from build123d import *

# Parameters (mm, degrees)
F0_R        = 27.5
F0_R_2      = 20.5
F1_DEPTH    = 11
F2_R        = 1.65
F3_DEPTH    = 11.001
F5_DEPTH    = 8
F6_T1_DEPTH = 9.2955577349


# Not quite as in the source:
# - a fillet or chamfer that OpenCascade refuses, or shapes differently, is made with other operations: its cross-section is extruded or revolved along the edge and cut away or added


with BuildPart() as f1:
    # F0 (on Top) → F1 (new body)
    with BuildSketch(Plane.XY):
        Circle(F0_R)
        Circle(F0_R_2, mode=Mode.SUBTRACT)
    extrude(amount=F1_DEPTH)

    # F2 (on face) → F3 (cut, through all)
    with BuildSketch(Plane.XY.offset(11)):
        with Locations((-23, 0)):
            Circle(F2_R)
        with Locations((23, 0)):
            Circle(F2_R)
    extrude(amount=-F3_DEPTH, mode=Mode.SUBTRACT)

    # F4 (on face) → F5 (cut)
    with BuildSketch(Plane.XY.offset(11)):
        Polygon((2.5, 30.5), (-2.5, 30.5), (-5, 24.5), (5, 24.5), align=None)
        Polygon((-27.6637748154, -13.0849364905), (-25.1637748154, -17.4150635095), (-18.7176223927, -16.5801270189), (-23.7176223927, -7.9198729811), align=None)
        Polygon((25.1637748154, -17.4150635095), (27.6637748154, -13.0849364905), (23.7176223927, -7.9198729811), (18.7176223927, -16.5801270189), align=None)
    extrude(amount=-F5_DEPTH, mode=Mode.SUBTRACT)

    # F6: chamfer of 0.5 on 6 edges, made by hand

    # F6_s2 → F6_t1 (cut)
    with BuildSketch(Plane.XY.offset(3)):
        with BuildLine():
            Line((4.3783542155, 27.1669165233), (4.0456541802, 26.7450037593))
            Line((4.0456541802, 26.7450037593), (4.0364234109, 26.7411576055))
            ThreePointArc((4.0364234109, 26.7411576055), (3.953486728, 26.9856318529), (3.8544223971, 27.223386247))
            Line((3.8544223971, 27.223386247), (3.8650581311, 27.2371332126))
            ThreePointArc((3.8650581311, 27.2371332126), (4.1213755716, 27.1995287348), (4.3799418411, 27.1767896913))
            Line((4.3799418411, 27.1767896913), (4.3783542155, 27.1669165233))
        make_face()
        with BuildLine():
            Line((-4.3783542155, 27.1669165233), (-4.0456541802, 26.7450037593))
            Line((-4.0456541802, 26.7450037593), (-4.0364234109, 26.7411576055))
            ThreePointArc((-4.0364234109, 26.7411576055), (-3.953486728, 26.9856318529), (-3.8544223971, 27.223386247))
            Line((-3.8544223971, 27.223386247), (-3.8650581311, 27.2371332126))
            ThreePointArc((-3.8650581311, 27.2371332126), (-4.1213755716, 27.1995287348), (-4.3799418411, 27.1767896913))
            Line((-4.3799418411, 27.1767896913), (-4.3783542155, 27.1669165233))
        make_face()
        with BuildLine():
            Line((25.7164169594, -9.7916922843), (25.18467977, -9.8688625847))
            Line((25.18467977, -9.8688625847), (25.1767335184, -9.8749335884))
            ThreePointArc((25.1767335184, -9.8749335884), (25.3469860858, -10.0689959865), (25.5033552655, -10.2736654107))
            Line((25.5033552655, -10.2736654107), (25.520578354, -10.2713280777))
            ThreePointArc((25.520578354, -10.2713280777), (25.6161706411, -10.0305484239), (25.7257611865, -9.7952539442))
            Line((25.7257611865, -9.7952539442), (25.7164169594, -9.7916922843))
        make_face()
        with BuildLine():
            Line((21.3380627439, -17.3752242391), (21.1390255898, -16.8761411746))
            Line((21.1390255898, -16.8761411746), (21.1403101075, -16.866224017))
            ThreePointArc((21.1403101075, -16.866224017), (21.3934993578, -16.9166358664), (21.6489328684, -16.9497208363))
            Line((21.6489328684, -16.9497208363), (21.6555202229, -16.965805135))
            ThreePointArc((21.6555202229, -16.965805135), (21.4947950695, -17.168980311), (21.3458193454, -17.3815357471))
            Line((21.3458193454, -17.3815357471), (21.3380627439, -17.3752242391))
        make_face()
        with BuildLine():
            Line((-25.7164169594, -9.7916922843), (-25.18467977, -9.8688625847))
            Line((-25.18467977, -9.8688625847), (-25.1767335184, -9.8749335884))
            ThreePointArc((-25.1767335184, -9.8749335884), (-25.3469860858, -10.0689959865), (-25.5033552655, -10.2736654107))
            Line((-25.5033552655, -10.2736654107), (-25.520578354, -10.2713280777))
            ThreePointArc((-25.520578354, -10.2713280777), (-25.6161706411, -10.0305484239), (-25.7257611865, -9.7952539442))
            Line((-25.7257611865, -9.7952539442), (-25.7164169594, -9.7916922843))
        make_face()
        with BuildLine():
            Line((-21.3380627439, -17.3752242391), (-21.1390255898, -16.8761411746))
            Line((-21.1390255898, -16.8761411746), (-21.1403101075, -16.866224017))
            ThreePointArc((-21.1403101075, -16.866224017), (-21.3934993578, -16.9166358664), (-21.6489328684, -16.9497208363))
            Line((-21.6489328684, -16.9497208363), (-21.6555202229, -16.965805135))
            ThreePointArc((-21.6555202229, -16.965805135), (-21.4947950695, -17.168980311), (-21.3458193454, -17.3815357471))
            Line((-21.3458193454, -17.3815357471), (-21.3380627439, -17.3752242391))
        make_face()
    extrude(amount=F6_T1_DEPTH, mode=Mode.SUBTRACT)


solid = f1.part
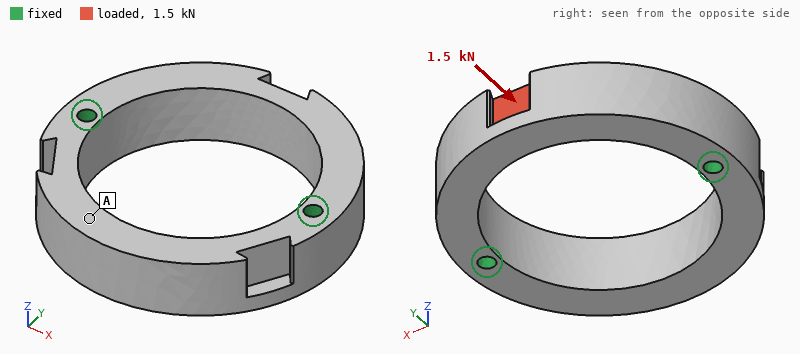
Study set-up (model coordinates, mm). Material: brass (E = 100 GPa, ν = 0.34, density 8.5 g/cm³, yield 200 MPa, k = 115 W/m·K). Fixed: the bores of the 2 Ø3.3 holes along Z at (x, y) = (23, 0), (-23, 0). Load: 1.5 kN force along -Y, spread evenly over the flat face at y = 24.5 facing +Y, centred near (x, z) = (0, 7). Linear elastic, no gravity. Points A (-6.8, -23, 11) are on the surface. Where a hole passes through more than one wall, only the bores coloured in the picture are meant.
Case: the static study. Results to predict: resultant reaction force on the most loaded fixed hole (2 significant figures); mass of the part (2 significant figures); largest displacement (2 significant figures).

1.0 kN
92 g
29 µm
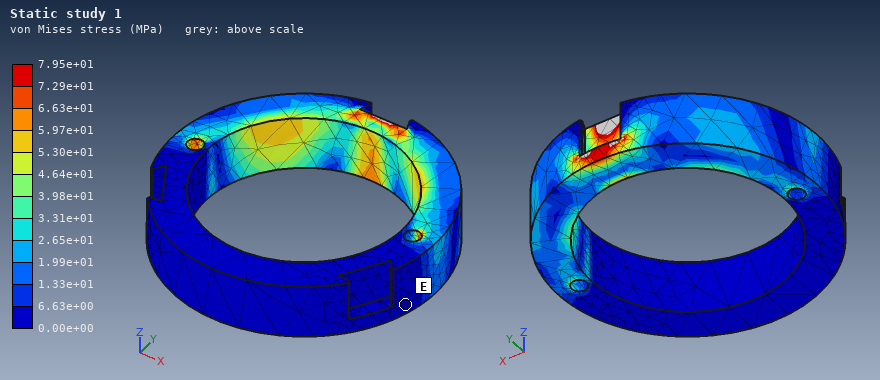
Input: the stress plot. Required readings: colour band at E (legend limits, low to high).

0.00e+00 to 6.63e+00 MPa
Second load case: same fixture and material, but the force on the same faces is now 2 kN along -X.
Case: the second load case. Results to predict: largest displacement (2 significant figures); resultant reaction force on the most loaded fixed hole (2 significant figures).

32 µm
1.2 kN
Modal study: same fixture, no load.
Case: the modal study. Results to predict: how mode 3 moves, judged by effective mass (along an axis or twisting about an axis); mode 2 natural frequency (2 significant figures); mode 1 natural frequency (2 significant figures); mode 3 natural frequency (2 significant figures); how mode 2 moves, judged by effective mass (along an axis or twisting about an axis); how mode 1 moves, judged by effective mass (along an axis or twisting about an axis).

twisting about Z
5200 Hz
4600 Hz
6700 Hz
along Z
along Z
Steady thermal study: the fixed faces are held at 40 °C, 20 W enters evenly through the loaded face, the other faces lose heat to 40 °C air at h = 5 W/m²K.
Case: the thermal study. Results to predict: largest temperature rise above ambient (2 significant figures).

44 K
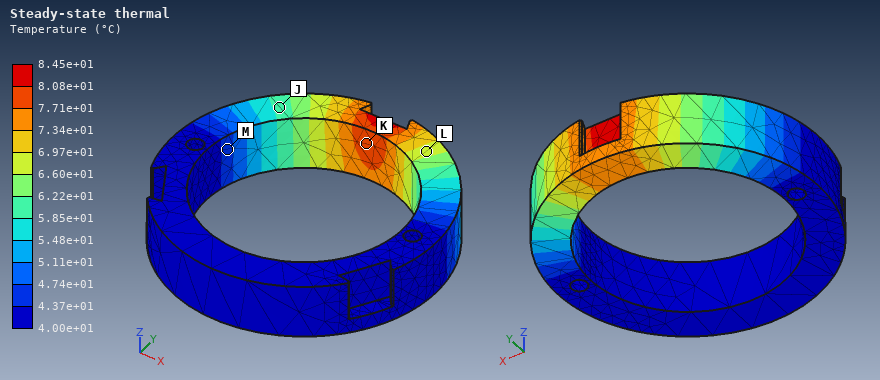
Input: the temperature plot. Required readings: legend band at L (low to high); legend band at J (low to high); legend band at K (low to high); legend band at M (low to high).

6.60e+01 to 6.97e+01 °C
5.85e+01 to 6.22e+01 °C
7.71e+01 to 8.08e+01 °C
4.37e+01 to 4.74e+01 °C
